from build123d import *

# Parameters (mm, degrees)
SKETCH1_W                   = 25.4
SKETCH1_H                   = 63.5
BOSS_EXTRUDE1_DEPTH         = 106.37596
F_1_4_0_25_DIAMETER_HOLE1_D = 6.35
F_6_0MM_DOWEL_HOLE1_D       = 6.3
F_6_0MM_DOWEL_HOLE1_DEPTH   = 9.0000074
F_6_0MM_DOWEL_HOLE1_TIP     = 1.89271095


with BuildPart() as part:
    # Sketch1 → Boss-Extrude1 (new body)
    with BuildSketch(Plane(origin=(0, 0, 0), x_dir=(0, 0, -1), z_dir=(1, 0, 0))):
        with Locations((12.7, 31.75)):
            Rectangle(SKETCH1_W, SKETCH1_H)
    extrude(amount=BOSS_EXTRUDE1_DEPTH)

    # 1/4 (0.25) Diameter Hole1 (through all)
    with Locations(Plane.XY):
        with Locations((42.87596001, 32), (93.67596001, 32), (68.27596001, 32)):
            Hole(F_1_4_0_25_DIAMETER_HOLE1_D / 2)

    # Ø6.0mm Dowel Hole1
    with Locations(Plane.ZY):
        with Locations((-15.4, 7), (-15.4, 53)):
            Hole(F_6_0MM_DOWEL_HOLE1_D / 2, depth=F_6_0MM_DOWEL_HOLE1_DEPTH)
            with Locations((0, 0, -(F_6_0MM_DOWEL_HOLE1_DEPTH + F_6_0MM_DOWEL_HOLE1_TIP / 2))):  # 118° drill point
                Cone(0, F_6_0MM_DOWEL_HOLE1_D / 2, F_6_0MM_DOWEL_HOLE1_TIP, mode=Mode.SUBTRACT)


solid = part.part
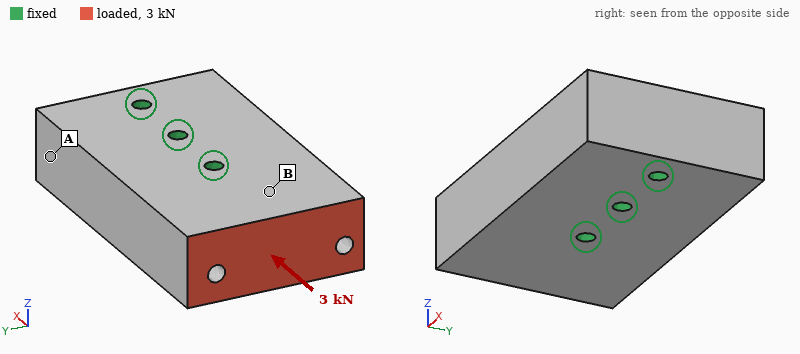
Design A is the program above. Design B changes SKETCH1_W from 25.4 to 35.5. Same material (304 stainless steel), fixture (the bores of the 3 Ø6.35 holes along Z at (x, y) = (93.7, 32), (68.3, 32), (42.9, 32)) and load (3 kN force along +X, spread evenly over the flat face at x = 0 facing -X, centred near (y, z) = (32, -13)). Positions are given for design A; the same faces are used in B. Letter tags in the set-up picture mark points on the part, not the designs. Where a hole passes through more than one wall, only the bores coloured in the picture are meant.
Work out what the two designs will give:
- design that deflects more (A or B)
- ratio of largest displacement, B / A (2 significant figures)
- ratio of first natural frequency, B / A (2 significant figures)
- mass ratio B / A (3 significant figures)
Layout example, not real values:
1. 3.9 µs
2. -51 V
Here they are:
1. A
2. 0.71
3. 1.2
4. 1.40
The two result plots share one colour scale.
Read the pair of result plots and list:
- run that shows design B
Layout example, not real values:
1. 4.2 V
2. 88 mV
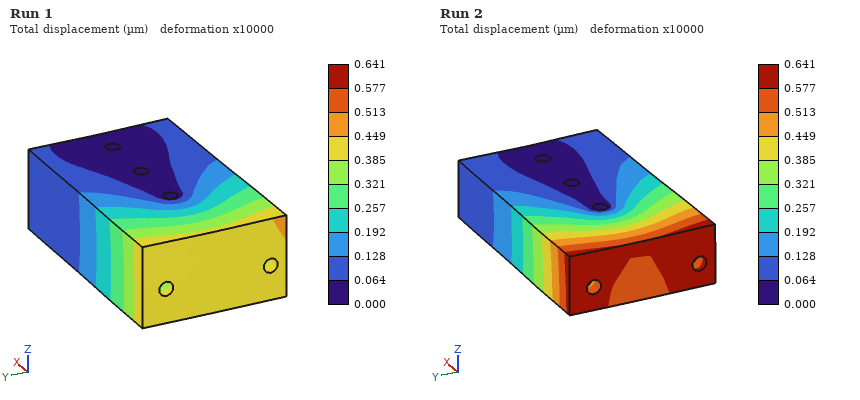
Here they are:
1. Run 1
